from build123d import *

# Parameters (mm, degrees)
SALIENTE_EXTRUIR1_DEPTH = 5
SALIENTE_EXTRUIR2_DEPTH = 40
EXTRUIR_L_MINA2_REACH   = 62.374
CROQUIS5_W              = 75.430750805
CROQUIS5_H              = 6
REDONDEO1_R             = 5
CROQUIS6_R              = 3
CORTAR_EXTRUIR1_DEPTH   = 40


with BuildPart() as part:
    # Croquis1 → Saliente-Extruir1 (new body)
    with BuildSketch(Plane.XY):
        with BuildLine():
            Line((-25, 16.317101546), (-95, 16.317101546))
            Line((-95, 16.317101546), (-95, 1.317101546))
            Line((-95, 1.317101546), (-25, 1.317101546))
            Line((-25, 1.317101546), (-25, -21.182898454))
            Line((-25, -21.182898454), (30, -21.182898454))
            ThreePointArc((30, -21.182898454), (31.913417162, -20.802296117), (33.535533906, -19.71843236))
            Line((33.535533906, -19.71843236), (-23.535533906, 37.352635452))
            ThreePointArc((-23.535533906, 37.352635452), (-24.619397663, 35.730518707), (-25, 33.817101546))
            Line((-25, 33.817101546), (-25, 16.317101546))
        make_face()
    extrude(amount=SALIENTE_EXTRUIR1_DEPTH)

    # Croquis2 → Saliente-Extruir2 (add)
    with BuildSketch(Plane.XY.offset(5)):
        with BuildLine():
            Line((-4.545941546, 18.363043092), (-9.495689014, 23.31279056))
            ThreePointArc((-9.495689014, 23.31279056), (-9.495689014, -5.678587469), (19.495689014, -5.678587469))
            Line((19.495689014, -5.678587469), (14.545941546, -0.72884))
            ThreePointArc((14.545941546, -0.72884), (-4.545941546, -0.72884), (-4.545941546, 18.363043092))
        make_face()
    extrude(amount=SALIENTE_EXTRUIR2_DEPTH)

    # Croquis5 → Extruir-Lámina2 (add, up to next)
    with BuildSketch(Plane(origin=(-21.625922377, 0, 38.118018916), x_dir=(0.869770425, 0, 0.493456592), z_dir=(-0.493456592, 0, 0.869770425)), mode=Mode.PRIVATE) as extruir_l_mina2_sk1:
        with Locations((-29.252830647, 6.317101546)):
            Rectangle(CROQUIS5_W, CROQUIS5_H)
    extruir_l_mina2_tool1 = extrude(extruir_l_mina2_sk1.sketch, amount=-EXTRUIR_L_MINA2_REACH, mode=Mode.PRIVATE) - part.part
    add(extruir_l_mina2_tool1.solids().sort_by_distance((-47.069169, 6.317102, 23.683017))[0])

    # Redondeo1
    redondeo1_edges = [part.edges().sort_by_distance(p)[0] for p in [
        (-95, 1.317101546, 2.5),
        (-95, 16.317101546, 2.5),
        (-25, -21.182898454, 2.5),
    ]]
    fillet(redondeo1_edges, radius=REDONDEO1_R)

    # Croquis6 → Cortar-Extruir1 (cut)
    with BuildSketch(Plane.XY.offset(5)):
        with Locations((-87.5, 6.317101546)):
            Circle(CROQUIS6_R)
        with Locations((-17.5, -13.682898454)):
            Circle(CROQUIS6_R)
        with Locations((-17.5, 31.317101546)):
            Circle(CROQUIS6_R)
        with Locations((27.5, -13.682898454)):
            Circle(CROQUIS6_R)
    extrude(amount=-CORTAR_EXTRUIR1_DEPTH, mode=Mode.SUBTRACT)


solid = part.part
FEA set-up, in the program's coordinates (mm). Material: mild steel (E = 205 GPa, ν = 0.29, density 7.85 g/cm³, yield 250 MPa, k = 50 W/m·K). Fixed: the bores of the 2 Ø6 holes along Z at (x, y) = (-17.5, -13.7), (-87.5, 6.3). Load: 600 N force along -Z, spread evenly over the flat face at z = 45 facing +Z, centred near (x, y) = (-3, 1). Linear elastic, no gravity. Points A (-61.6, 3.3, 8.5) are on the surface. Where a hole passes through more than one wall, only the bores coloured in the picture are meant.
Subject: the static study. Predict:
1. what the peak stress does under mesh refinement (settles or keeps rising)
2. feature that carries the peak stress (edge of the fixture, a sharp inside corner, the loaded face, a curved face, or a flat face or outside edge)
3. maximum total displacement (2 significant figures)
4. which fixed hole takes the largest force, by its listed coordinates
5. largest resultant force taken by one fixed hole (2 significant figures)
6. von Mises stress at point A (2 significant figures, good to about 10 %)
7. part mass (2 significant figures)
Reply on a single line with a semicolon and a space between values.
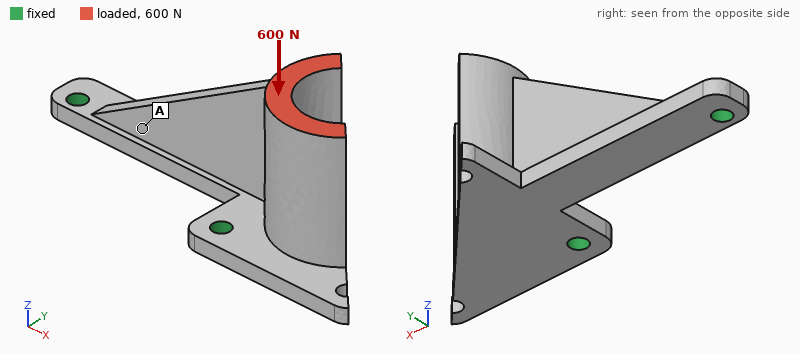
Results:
keeps rising; edge of the fixture; 56 µm; (-17.5, -13.7); 680 N; 12 MPa; 280 g
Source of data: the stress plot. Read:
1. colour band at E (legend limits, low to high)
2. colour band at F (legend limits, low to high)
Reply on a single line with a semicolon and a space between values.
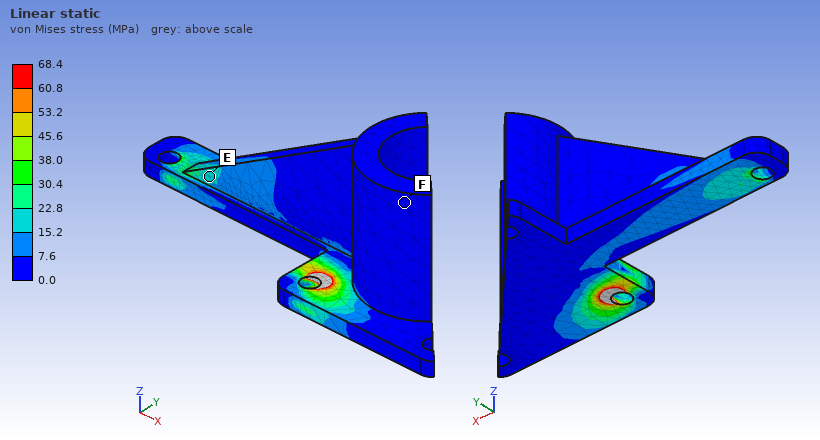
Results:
15.2 to 22.8 MPa; 0.0 to 7.6 MPa
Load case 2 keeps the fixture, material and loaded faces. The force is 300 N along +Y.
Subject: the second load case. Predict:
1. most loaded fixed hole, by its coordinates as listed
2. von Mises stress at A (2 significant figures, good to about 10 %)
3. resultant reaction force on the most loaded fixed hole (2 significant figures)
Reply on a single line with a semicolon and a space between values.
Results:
(-17.5, -13.7); 20 MPa; 320 N
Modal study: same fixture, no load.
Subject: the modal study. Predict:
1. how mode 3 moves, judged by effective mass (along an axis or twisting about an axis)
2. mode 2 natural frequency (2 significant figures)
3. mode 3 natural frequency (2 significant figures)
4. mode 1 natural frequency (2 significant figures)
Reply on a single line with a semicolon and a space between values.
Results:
along Z; 3500 Hz; 4700 Hz; 1100 Hz
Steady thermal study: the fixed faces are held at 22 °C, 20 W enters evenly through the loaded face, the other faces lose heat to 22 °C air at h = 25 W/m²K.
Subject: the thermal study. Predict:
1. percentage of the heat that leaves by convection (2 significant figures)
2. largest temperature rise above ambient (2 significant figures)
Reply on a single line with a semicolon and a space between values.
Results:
41 %; 56 K
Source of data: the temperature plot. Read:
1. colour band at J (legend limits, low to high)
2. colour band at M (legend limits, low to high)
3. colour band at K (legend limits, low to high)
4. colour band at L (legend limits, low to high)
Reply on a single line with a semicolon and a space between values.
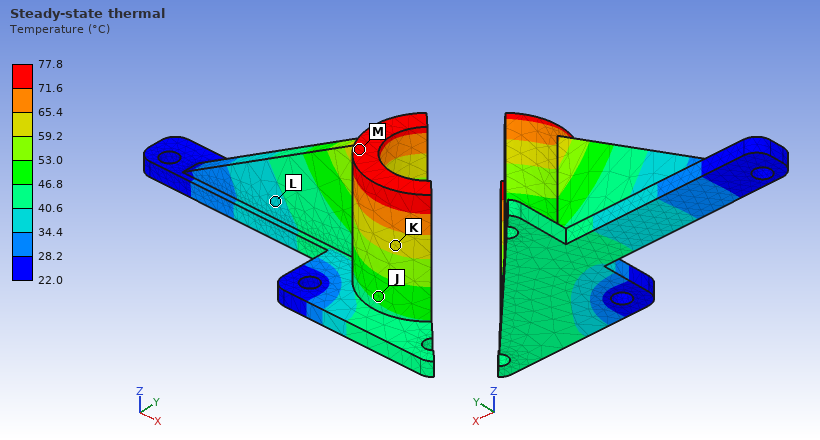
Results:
46.8 to 53.0 °C; 71.6 to 77.8 °C; 59.2 to 65.4 °C; 34.4 to 40.6 °C
